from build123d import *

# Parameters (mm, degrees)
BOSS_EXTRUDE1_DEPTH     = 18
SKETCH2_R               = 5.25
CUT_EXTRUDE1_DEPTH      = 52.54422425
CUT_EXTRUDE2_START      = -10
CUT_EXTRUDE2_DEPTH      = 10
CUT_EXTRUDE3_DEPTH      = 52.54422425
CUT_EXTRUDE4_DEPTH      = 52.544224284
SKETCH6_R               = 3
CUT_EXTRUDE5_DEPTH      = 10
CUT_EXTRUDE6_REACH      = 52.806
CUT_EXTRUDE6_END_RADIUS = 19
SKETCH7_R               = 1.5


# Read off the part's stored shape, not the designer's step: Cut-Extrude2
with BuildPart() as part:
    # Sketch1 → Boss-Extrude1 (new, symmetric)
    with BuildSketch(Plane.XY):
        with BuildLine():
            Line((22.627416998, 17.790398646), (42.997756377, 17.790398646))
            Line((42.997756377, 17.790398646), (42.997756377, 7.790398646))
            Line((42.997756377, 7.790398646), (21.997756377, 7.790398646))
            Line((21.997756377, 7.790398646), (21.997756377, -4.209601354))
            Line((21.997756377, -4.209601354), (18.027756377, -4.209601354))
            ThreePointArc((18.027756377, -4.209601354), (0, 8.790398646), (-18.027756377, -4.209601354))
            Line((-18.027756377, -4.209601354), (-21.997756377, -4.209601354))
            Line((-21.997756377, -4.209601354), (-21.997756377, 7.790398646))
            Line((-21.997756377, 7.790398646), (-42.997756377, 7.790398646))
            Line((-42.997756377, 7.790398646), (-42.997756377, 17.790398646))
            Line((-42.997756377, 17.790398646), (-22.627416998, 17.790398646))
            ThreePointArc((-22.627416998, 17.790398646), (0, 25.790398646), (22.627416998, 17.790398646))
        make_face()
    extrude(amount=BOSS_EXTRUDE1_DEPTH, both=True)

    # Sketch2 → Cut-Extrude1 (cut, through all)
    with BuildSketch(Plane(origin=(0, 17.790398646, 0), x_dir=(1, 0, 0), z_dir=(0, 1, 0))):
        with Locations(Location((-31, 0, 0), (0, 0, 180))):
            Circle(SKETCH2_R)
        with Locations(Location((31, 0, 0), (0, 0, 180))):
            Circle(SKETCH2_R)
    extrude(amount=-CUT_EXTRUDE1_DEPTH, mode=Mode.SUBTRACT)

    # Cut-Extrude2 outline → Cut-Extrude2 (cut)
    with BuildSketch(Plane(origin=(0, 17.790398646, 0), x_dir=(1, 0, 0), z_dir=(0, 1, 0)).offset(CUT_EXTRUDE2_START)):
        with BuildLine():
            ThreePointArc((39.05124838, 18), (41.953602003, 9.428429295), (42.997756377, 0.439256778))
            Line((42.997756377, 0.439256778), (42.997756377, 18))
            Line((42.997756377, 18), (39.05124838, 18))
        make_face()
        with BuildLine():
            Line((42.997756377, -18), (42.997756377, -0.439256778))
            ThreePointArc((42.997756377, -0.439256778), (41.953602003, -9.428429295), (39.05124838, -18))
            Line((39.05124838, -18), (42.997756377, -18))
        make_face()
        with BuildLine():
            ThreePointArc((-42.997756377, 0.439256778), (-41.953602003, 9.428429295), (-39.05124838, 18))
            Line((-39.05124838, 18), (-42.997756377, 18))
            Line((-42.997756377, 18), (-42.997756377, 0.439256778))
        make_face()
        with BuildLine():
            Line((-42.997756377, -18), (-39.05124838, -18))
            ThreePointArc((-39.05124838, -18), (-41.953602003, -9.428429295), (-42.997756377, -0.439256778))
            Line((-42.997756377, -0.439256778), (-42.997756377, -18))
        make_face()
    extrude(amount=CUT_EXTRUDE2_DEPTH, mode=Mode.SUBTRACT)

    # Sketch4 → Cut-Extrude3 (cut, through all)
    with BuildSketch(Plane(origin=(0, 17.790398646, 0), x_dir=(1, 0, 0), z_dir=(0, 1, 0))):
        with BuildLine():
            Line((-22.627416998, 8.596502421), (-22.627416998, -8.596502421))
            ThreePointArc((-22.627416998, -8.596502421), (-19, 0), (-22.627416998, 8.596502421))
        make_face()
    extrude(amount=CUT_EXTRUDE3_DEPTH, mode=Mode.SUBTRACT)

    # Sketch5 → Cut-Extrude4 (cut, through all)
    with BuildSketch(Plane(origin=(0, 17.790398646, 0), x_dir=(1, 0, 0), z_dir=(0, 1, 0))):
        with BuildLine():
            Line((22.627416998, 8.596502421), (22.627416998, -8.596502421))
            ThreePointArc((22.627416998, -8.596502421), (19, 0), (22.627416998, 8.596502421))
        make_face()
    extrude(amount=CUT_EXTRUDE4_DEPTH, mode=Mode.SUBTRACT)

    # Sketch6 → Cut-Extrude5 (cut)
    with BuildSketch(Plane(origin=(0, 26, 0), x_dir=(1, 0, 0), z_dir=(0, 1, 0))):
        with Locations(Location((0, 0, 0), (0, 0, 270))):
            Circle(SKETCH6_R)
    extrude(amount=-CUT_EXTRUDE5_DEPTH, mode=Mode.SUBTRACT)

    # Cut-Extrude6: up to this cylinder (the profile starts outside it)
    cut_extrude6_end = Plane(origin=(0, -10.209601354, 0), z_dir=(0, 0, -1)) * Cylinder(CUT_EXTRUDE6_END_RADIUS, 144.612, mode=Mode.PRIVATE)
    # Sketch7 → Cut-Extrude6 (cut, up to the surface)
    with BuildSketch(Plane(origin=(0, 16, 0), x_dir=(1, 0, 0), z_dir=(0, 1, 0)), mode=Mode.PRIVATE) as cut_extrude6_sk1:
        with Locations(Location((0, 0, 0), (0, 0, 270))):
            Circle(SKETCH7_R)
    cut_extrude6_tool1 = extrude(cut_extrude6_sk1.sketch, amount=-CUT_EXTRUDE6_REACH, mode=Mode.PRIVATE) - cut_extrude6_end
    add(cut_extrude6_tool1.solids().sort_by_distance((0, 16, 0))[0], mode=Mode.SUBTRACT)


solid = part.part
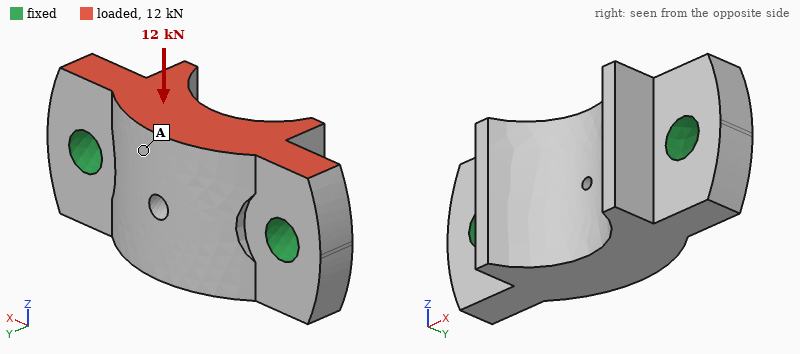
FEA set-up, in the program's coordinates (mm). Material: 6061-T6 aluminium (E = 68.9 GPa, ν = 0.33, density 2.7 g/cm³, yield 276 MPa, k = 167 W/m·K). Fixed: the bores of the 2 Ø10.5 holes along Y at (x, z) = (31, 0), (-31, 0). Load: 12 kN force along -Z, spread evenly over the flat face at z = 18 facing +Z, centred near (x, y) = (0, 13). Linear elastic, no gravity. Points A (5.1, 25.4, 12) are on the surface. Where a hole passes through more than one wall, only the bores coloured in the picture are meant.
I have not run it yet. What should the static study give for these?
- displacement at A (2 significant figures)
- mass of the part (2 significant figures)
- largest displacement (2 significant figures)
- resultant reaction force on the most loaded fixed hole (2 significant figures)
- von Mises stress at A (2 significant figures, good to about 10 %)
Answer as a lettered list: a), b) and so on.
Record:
a) 16 µm
b) 120 g
c) 17 µm
d) 6.0 kN
e) 9.0 MPa
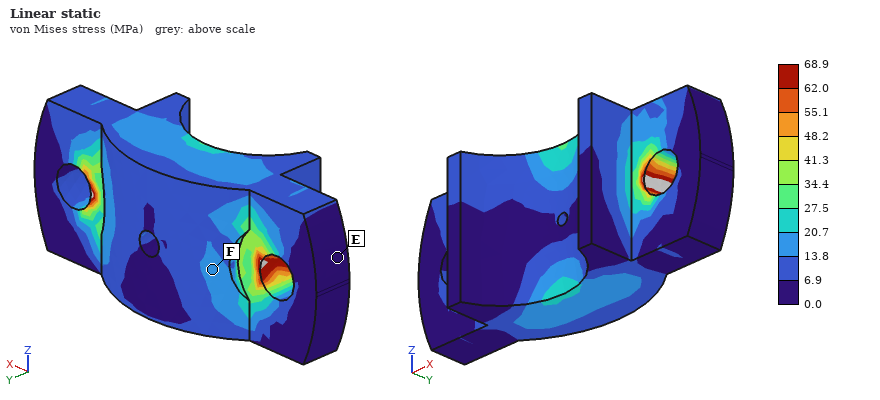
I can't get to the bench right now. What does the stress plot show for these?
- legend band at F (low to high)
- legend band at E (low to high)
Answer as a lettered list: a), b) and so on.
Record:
a) 13.8 to 20.7 MPa
b) 0.0 to 6.9 MPa
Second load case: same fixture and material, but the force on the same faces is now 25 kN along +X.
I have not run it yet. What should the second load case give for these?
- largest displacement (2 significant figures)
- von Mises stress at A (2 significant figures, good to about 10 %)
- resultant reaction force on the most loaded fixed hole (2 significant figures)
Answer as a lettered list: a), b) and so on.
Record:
a) 41 µm
b) 19 MPa
c) 14 kN
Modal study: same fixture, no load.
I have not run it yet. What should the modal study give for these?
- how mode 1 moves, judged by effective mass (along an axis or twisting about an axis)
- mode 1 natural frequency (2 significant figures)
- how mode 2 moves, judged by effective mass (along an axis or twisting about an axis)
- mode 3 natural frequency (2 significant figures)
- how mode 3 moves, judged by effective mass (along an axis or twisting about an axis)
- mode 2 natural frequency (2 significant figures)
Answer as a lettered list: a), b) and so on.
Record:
a) twisting about X
b) 11 kHz
c) along Y
d) 16 kHz
e) along Z
f) 12 kHz
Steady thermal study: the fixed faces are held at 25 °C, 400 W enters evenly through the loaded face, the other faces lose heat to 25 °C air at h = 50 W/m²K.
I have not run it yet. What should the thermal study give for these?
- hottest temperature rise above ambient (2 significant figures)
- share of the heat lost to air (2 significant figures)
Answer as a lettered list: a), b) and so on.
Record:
a) 65 K
b) 3.0 %
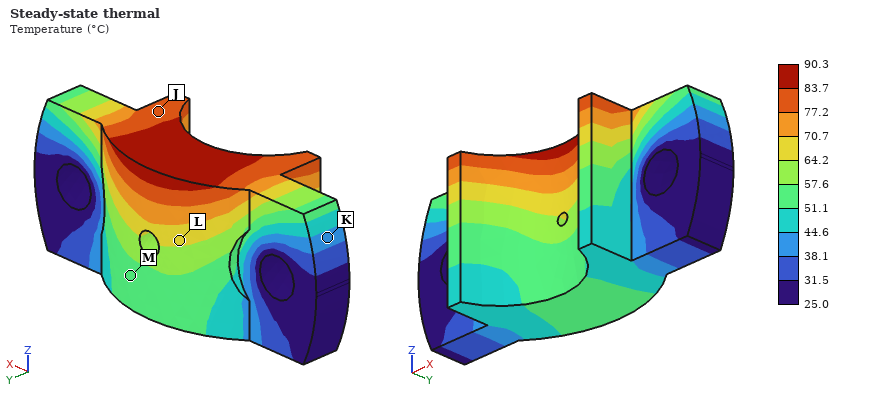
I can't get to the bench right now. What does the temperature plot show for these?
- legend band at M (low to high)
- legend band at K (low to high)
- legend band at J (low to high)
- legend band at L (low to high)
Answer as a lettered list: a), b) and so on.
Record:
a) 51.1 to 57.6 °C
b) 38.1 to 44.6 °C
c) 77.2 to 83.7 °C
d) 64.2 to 70.7 °C
